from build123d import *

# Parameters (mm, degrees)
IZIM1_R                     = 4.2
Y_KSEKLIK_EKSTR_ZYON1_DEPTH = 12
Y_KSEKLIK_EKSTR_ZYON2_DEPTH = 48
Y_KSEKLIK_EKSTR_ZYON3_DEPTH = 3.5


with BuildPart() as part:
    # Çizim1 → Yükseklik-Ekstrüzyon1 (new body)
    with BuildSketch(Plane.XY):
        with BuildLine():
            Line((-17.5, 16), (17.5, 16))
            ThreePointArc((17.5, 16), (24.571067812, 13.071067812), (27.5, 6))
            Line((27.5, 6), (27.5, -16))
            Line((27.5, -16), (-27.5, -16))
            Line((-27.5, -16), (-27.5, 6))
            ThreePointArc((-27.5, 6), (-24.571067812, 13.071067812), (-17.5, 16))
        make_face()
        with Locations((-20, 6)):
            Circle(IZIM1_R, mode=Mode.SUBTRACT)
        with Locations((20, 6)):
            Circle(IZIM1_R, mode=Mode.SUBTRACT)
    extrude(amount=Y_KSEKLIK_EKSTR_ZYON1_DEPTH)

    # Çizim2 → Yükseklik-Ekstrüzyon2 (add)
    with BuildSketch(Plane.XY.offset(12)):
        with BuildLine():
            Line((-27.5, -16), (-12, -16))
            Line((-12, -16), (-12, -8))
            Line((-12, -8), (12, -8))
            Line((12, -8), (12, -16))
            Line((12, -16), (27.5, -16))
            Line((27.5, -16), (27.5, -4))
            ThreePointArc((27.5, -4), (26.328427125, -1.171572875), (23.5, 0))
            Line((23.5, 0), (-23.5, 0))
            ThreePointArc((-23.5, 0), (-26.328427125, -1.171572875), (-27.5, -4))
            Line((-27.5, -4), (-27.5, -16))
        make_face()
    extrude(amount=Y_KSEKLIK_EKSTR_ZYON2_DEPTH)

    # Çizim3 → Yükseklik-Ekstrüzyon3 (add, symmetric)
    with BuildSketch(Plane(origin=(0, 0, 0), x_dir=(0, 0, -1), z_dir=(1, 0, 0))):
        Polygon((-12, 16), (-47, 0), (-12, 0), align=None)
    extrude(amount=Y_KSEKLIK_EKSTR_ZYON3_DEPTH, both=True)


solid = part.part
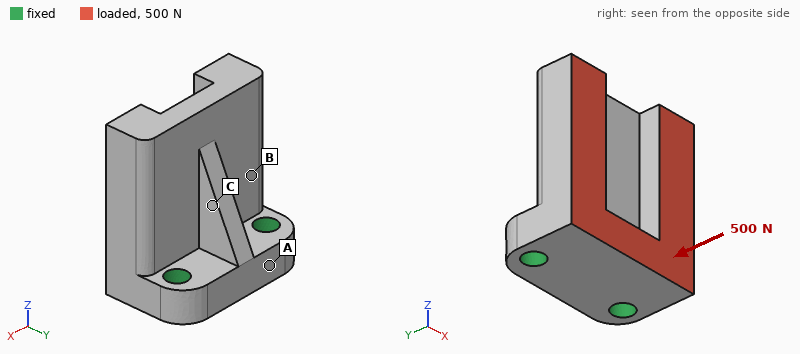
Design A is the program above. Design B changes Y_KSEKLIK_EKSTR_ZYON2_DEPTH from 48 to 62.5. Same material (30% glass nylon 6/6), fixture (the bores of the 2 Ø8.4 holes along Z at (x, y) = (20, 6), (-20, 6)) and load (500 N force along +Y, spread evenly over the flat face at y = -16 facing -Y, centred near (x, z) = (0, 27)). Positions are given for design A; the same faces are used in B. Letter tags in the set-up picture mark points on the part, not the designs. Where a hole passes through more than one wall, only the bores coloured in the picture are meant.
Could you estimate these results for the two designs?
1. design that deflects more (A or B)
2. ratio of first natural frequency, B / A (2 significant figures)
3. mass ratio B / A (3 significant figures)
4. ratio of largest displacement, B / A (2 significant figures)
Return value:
B
0.68
1.18
1.8
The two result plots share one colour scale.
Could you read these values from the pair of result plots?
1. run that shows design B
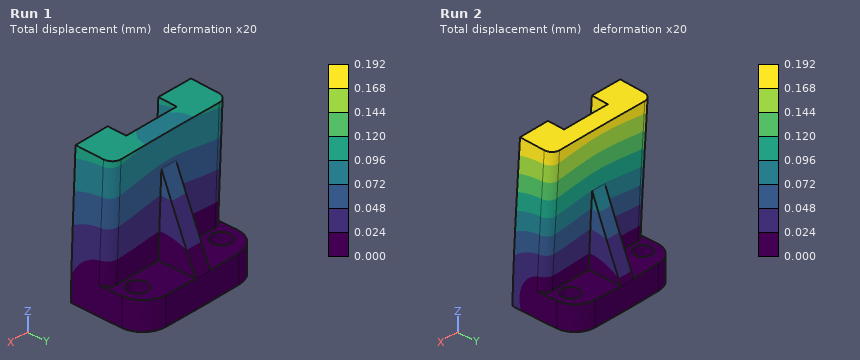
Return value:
Run 2
